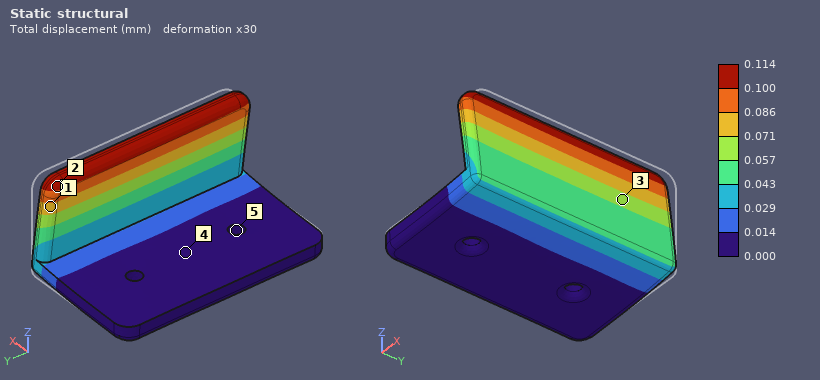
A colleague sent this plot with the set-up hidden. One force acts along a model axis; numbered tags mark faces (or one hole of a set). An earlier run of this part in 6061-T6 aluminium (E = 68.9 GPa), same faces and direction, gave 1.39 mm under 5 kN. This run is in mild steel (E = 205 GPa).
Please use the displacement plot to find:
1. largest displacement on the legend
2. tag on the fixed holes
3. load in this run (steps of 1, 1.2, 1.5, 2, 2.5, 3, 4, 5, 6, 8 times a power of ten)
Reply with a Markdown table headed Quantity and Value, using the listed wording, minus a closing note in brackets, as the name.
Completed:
| Quantity | Value |
|---|---|
| largest displacement on the legend | 0.114 mm |
| tag on the fixed holes | 5 |
| load in this run | 1.2 kN |
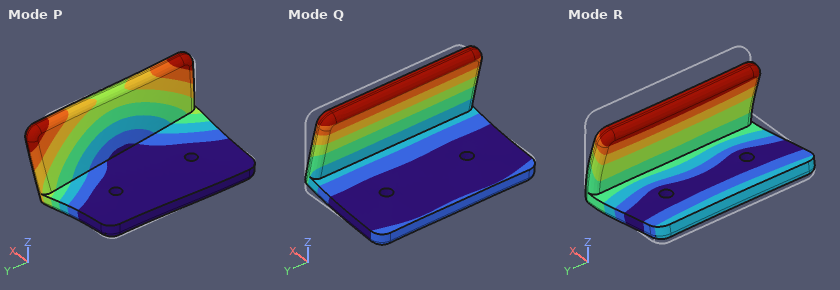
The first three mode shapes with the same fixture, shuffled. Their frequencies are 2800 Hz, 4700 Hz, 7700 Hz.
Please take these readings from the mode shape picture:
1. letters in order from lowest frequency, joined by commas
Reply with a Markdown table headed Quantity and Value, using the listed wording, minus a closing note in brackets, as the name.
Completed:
| Quantity | Value |
|---|---|
| letters in order from lowest frequency, joined by commas | Q, P, R |
